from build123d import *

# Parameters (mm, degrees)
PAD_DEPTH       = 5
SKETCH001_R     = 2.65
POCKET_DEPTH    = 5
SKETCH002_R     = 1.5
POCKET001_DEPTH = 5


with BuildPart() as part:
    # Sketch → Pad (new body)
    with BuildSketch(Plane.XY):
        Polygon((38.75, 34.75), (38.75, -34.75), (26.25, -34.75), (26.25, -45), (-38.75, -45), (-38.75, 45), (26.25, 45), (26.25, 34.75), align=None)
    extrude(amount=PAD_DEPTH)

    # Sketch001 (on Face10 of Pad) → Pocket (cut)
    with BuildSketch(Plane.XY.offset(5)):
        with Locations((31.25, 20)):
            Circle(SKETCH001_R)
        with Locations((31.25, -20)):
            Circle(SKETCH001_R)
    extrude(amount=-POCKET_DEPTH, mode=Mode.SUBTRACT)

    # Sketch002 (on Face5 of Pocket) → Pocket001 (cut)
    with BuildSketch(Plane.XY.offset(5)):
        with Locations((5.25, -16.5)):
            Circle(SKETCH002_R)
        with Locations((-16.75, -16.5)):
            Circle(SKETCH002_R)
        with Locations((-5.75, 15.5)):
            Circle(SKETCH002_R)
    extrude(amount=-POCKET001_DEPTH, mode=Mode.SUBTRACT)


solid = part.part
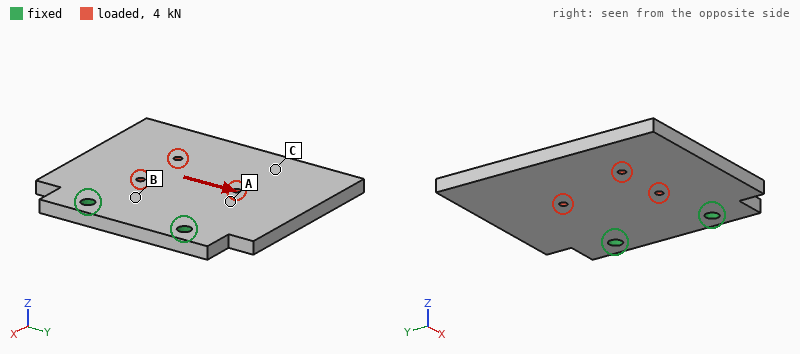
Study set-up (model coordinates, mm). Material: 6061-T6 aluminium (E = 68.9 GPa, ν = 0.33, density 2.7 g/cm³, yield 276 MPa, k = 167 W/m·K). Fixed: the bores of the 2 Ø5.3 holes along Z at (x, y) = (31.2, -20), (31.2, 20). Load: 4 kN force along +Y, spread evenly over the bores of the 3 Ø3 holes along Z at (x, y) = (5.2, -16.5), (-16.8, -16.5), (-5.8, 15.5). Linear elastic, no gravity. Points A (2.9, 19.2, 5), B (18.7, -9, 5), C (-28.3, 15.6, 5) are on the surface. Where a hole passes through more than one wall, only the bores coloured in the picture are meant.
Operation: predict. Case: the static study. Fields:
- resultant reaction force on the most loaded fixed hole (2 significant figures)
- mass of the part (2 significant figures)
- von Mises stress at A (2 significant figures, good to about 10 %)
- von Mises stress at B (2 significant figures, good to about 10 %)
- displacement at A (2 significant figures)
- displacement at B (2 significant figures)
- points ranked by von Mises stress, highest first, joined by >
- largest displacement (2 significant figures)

3.9 kN
90 g
19 MPa
35 MPa
28 µm
12 µm
B > A > C
62 µm
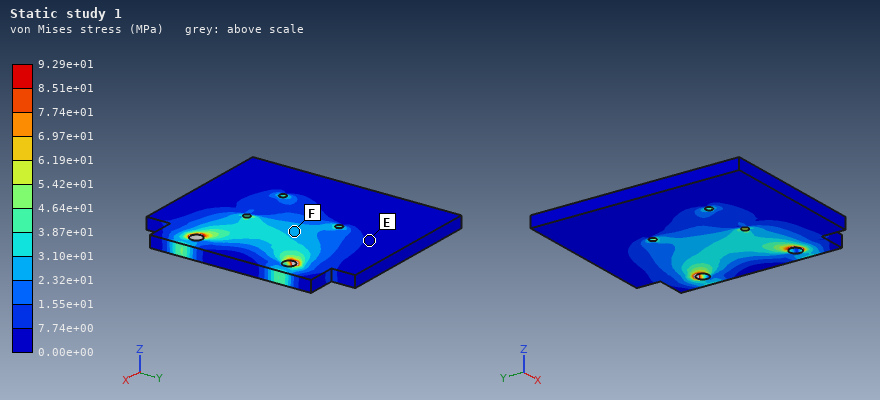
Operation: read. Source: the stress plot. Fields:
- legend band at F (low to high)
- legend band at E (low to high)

2.32e+01 to 3.10e+01 MPa
0.00e+00 to 7.74e+00 MPa
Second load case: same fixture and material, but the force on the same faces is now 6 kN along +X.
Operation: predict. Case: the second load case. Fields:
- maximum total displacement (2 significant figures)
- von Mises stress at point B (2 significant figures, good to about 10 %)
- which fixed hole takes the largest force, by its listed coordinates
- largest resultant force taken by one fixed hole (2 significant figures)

20 µm
20 MPa
(31.2, -20)
3.8 kN
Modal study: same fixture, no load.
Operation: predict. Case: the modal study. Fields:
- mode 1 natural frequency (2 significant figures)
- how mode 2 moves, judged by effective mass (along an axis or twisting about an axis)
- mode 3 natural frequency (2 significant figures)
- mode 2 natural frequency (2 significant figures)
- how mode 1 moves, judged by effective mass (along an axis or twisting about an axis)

760 Hz
twisting about X
3600 Hz
1500 Hz
along Z
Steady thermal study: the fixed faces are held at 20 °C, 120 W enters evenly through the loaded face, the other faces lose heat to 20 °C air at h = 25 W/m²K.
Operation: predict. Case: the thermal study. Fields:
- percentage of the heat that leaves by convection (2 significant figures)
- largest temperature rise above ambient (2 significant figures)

14 %
83 K
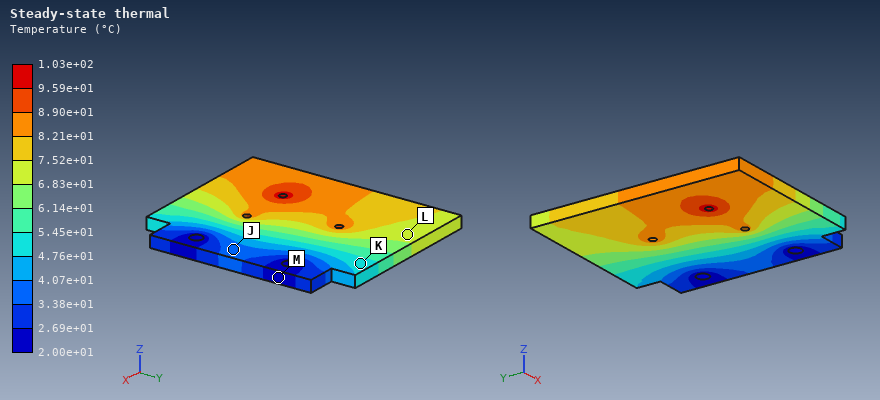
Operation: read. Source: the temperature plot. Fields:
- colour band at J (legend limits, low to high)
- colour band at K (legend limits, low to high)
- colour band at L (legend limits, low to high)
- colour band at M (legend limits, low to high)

3.38e+01 to 4.07e+01 °C
4.76e+01 to 5.45e+01 °C
6.83e+01 to 7.52e+01 °C
2.00e+01 to 2.69e+01 °C
